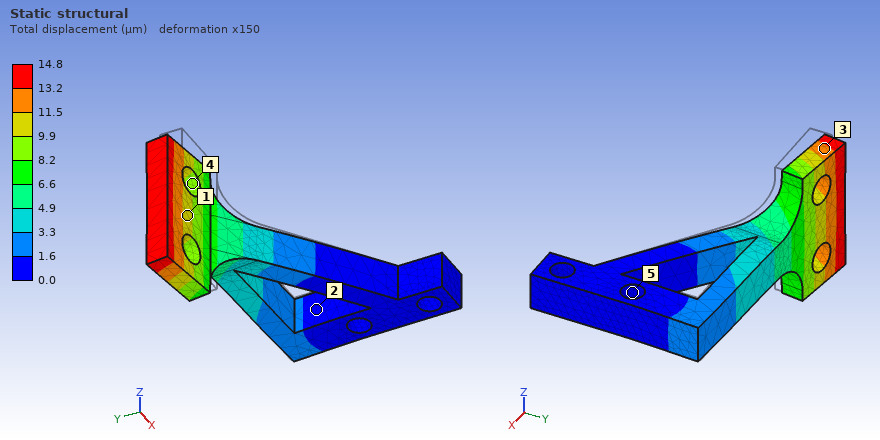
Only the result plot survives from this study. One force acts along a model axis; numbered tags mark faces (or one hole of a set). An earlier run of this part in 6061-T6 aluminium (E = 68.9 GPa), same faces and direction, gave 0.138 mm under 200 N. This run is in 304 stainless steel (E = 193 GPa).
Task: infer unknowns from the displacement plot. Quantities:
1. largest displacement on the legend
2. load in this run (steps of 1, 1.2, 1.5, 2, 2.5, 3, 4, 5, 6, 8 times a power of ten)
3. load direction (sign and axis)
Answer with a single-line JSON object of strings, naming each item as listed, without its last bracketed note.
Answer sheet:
{"largest displacement on the legend": "14.8 µm", "load in this run": "60 N", "load direction": "+Y"}
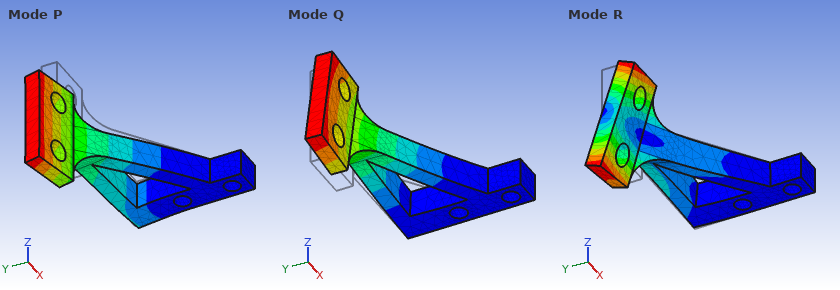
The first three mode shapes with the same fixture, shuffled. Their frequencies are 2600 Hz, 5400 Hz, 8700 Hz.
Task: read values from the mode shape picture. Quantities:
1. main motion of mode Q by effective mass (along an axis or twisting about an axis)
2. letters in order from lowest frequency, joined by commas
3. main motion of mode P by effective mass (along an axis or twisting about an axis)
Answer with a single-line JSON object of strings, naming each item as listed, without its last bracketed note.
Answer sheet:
{"main motion of mode Q by effective mass": "along Z", "letters in order from lowest frequency, joined by commas": "Q, P, R", "main motion of mode P by effective mass": "along Y"}
